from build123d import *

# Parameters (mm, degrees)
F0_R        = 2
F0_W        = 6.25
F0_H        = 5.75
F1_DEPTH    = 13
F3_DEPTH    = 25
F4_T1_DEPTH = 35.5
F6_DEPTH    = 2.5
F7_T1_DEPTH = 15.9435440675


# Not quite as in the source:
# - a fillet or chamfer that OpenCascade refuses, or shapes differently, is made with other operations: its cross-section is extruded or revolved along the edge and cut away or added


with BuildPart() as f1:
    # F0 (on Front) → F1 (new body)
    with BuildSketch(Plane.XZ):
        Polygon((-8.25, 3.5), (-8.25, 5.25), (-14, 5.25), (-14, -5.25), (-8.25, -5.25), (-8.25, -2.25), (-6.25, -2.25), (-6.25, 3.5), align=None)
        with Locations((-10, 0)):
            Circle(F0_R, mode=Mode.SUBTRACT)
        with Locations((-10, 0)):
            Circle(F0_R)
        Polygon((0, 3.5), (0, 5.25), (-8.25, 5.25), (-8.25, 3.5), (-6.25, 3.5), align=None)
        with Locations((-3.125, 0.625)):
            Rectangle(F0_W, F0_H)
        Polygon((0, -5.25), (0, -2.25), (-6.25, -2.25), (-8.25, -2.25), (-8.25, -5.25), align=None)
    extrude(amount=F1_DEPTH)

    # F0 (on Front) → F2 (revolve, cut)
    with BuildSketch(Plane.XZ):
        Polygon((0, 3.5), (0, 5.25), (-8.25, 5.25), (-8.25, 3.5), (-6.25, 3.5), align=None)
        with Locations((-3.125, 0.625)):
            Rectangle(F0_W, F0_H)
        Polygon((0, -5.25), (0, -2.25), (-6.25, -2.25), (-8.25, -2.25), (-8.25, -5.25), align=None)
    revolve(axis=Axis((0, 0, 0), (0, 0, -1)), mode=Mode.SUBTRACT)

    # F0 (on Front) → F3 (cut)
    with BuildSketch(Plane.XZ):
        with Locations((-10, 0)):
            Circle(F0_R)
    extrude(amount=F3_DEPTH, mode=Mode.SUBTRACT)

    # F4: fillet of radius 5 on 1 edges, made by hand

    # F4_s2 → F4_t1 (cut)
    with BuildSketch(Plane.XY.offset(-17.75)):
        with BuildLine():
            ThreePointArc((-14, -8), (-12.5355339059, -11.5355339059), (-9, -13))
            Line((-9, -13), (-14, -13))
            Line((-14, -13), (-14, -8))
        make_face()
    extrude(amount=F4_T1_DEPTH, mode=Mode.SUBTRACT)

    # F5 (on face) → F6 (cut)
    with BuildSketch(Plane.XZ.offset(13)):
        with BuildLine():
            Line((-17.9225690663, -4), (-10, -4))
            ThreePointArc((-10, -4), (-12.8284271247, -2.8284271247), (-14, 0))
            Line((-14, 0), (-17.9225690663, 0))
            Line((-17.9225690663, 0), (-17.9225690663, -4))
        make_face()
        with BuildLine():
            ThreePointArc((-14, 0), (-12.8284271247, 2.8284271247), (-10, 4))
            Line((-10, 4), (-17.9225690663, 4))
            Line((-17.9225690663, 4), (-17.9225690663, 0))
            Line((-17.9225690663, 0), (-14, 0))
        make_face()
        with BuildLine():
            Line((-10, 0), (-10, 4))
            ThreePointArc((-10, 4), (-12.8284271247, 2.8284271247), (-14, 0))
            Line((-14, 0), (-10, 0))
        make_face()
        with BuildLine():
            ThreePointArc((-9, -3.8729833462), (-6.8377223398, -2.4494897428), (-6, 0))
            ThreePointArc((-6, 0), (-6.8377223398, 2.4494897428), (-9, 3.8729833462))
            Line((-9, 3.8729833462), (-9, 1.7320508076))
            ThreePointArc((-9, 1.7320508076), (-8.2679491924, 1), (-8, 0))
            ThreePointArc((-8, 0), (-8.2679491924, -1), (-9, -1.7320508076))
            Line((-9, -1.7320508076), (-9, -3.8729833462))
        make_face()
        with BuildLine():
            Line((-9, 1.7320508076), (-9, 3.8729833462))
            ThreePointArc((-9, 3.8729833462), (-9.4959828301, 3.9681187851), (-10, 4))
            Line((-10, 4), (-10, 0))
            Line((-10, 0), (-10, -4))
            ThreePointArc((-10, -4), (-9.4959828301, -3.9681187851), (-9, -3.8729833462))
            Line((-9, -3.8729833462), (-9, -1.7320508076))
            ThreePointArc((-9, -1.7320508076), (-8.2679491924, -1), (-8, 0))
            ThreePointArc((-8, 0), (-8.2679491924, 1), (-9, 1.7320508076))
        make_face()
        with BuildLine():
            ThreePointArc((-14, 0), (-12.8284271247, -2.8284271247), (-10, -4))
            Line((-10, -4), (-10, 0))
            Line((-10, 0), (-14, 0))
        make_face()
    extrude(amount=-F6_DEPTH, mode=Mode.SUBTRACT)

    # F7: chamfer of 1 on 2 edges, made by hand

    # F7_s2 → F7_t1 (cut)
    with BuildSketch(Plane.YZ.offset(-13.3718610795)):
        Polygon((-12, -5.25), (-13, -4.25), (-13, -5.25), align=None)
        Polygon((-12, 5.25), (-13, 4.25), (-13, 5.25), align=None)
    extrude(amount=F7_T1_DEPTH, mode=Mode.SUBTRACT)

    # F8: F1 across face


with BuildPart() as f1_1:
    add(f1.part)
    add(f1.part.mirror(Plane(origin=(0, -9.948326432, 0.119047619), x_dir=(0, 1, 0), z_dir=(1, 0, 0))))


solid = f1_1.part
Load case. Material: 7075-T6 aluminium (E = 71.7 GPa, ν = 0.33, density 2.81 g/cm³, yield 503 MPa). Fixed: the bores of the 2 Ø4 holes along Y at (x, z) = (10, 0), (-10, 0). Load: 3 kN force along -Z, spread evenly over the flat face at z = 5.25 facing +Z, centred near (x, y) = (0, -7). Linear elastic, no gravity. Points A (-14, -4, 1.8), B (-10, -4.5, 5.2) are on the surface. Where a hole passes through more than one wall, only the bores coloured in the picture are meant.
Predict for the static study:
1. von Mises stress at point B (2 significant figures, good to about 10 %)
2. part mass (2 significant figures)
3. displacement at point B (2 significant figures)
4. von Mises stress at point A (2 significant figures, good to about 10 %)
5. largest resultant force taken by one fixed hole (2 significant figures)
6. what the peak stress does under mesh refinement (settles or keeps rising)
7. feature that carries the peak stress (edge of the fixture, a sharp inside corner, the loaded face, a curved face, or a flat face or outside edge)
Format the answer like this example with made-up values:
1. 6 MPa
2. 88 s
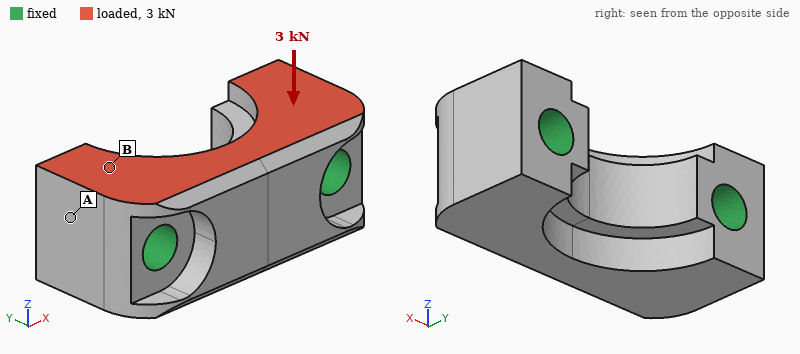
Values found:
1. 20 MPa
2. 6.6 g
3. 0.76 µm
4. 7.4 MPa
5. 1.5 kN
6. keeps rising
7. edge of the fixture
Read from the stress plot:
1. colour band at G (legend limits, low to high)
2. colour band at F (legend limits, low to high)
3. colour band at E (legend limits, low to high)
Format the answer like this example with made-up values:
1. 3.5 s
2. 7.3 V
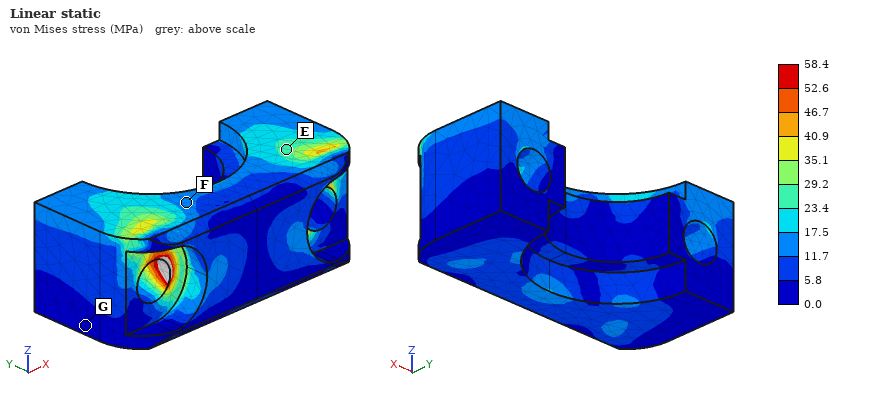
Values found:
1. 0.0 to 5.8 MPa
2. 11.7 to 17.5 MPa
3. 23.4 to 29.2 MPa
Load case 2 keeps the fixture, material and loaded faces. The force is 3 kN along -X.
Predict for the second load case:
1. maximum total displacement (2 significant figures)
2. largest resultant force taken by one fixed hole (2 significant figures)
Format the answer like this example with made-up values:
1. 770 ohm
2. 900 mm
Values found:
1. 4.9 µm
2. 1.6 kN
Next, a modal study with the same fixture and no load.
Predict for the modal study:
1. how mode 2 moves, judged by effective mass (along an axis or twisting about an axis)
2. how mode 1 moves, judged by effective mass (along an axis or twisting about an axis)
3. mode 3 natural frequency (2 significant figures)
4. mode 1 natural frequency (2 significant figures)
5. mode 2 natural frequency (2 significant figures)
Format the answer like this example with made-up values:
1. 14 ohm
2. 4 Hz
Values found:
1. along Y
2. along Z
3. 88 kHz
4. 55 kHz
5. 74 kHz
